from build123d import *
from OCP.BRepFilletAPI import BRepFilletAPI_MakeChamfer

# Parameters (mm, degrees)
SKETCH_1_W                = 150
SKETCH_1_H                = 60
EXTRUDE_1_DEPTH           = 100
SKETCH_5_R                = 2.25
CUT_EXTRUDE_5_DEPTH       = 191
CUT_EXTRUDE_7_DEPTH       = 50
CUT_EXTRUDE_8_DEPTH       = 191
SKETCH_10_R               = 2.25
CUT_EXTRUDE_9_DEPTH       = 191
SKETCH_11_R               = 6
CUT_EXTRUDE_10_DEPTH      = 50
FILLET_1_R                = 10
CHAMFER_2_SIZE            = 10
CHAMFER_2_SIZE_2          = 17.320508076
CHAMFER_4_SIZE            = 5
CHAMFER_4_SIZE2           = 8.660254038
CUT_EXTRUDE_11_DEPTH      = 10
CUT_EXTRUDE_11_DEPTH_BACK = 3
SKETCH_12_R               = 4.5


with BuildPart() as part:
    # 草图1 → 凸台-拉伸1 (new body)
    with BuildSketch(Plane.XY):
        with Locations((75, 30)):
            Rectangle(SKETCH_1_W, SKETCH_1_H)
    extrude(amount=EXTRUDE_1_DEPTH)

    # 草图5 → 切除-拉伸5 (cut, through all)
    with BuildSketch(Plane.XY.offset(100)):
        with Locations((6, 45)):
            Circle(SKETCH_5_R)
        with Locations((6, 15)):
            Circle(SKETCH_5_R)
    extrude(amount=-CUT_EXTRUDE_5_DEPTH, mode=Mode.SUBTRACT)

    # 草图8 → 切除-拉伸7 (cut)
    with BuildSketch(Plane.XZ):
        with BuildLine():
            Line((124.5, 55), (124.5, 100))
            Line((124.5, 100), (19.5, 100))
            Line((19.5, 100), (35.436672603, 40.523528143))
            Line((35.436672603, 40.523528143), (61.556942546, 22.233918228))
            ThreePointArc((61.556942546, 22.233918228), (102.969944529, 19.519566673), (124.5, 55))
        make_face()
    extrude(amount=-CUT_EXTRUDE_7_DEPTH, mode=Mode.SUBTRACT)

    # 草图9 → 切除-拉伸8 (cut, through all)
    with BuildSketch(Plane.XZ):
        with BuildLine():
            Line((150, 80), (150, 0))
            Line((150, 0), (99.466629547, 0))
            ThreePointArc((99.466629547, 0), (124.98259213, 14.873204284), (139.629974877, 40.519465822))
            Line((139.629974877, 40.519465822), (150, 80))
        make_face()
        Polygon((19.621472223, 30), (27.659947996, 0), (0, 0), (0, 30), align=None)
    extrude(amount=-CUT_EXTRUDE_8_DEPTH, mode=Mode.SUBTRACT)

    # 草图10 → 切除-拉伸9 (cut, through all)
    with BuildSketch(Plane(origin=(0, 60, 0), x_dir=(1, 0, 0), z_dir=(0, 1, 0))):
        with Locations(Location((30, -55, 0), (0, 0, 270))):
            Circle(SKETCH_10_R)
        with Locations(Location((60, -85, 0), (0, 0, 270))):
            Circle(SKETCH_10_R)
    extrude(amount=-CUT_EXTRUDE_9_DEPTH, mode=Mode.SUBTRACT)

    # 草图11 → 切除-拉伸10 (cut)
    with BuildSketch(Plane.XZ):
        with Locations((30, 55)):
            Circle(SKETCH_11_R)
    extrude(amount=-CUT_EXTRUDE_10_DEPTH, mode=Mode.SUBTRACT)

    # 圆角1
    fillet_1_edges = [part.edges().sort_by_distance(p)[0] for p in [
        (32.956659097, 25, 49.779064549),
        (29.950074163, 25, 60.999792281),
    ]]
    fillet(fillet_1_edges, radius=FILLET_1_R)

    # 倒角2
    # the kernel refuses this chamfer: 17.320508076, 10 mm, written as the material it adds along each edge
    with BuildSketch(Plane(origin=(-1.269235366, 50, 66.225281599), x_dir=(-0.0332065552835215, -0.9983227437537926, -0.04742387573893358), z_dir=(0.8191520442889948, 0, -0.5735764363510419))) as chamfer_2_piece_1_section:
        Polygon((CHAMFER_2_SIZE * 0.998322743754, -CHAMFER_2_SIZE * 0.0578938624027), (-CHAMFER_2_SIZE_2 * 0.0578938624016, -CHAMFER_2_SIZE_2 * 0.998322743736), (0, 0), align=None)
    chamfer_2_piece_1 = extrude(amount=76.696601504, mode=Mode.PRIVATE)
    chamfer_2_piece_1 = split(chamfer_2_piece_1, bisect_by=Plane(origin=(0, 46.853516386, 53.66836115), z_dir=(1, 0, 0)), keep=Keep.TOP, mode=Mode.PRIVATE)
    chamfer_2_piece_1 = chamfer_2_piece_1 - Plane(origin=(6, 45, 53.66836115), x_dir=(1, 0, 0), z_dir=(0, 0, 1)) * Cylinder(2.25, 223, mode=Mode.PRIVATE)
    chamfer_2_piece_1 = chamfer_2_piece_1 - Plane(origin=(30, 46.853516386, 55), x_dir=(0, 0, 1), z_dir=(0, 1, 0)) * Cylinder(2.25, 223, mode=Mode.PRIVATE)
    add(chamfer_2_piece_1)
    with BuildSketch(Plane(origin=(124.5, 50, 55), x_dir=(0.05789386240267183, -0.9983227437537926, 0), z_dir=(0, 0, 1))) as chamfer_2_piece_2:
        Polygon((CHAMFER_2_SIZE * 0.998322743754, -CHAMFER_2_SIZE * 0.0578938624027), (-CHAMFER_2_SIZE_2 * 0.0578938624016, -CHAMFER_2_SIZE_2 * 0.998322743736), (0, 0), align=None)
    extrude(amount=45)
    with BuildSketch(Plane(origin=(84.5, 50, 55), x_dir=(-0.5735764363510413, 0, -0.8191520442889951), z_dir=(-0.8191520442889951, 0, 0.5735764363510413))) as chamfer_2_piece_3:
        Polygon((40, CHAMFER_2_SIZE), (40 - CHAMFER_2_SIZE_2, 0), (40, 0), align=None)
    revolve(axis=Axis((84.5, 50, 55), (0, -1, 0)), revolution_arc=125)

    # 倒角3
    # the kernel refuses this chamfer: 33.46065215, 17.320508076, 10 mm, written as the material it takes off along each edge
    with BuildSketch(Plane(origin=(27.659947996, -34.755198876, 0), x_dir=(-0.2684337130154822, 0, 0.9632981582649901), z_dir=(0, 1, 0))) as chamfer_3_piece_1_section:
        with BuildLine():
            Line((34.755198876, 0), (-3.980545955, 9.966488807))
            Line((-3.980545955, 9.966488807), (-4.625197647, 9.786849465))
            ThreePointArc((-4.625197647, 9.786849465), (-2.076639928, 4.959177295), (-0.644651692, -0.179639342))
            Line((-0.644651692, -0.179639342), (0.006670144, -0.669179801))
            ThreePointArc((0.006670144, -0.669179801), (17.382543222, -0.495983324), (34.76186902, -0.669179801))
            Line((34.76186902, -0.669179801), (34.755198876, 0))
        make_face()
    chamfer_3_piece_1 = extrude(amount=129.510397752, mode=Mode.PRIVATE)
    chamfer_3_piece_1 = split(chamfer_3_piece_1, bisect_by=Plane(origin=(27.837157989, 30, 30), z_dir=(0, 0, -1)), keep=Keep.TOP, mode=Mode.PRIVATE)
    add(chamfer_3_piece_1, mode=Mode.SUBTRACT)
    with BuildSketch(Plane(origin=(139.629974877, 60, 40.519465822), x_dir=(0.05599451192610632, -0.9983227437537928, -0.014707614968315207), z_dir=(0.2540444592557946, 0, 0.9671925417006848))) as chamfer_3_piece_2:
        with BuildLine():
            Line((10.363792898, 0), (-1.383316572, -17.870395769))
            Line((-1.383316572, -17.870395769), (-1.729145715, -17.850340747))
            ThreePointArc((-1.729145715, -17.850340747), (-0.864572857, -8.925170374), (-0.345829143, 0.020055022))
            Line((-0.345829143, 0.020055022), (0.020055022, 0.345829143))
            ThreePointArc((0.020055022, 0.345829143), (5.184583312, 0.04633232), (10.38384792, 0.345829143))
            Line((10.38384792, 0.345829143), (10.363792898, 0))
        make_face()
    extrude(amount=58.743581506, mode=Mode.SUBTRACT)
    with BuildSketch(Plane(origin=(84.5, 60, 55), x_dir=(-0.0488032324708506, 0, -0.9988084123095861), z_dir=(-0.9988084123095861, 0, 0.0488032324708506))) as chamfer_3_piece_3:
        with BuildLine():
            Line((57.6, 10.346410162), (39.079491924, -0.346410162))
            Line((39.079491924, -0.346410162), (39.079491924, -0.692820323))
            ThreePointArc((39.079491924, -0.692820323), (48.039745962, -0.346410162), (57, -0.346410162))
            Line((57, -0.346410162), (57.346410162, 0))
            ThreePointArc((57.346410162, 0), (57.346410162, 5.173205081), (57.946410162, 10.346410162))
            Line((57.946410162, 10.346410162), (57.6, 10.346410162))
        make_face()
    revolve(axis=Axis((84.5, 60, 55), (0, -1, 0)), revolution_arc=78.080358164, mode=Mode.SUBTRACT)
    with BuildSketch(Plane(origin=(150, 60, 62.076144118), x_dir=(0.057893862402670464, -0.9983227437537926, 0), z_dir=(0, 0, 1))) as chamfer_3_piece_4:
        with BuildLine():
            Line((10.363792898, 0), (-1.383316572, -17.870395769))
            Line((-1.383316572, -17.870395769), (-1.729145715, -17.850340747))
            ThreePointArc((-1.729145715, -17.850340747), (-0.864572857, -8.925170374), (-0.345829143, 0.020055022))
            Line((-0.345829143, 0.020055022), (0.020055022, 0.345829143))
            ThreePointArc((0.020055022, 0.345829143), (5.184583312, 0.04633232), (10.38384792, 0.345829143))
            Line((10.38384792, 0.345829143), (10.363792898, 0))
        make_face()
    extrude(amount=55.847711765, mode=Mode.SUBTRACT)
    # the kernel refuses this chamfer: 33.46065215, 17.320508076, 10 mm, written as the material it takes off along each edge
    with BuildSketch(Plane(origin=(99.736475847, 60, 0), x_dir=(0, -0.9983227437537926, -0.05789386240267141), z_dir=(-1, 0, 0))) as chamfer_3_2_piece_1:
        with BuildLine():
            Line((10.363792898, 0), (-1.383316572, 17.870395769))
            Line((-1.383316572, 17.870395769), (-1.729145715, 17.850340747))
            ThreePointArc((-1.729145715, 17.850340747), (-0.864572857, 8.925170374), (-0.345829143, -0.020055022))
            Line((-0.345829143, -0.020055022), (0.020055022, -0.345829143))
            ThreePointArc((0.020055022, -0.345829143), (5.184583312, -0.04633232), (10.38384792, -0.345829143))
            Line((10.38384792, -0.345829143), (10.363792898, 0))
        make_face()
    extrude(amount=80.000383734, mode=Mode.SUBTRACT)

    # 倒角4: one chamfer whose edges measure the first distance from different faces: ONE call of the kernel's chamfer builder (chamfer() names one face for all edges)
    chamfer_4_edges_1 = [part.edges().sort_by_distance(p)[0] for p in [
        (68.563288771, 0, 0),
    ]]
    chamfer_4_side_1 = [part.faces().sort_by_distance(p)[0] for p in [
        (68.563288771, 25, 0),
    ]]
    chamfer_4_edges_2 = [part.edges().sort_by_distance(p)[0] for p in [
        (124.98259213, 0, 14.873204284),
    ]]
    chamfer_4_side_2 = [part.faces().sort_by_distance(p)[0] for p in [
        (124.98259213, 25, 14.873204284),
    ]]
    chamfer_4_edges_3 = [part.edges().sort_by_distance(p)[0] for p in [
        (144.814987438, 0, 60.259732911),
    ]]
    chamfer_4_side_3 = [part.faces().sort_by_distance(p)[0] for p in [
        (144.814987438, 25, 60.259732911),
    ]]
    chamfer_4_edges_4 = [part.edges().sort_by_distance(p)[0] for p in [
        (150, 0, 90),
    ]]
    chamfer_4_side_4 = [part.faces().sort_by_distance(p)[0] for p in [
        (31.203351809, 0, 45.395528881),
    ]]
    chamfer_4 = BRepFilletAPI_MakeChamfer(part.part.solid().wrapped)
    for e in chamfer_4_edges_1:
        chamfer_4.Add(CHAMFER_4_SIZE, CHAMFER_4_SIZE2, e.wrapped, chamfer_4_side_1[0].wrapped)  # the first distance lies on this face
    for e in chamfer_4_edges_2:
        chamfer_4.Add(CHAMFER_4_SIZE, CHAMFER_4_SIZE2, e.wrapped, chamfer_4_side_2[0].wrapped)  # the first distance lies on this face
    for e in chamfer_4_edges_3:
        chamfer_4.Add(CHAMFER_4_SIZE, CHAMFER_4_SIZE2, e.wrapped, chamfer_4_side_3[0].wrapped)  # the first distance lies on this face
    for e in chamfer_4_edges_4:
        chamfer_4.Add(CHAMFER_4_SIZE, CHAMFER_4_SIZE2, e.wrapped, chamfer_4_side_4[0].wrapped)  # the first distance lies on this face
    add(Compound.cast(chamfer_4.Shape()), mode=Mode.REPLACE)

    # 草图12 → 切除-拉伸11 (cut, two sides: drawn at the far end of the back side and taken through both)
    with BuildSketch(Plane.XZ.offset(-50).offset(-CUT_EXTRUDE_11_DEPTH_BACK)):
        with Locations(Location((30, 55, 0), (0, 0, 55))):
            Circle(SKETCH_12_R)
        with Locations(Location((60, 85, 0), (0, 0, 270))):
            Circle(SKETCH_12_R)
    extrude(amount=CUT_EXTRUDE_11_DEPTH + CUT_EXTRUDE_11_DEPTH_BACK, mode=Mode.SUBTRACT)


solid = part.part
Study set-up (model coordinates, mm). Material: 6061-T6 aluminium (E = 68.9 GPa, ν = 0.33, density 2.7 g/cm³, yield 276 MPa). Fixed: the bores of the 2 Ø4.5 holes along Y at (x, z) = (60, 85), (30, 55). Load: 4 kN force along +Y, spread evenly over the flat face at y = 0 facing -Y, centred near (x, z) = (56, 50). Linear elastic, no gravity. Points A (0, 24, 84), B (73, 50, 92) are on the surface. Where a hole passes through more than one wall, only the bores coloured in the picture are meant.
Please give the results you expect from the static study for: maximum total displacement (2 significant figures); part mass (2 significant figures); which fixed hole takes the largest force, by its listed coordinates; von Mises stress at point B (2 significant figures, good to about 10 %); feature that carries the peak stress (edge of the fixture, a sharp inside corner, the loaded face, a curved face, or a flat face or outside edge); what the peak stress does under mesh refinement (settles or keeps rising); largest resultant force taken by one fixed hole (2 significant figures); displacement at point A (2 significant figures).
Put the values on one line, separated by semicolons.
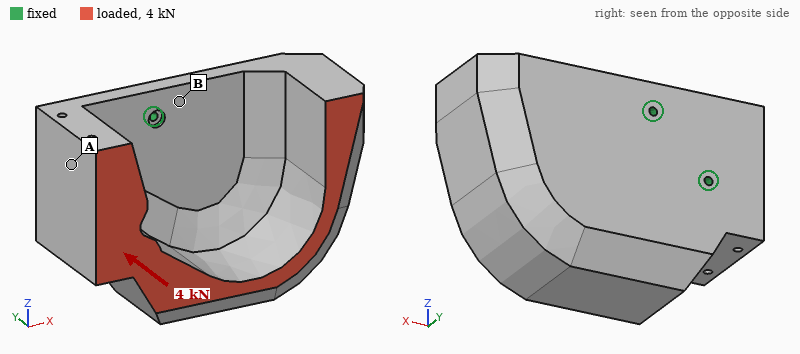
0.43 mm; 1.1 kg; (30, 55); 30 MPa; edge of the fixture; keeps rising; 2.6 kN; 0.18 mm
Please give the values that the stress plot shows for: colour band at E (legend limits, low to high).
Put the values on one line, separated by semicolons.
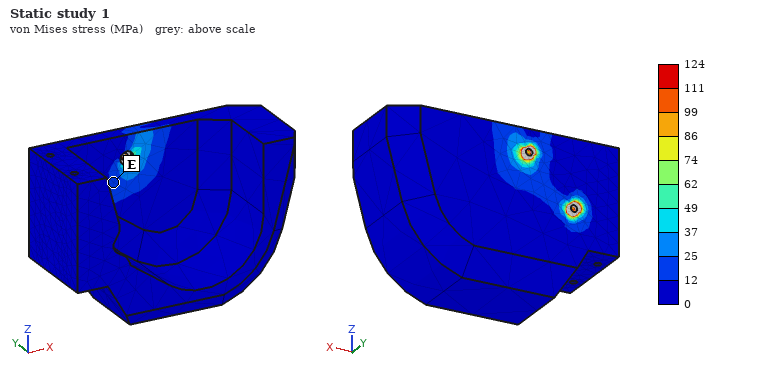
12 to 25 MPa
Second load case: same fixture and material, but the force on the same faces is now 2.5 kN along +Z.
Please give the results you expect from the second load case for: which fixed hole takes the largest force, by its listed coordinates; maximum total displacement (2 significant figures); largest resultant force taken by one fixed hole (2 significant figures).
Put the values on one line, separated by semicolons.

(60, 85); 0.48 mm; 2.8 kN
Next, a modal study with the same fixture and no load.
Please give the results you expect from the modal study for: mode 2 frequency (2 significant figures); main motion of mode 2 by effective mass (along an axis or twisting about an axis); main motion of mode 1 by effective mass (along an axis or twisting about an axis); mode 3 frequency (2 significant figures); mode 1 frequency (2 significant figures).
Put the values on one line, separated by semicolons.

950 Hz; along Z; along Y; 1700 Hz; 390 Hz
